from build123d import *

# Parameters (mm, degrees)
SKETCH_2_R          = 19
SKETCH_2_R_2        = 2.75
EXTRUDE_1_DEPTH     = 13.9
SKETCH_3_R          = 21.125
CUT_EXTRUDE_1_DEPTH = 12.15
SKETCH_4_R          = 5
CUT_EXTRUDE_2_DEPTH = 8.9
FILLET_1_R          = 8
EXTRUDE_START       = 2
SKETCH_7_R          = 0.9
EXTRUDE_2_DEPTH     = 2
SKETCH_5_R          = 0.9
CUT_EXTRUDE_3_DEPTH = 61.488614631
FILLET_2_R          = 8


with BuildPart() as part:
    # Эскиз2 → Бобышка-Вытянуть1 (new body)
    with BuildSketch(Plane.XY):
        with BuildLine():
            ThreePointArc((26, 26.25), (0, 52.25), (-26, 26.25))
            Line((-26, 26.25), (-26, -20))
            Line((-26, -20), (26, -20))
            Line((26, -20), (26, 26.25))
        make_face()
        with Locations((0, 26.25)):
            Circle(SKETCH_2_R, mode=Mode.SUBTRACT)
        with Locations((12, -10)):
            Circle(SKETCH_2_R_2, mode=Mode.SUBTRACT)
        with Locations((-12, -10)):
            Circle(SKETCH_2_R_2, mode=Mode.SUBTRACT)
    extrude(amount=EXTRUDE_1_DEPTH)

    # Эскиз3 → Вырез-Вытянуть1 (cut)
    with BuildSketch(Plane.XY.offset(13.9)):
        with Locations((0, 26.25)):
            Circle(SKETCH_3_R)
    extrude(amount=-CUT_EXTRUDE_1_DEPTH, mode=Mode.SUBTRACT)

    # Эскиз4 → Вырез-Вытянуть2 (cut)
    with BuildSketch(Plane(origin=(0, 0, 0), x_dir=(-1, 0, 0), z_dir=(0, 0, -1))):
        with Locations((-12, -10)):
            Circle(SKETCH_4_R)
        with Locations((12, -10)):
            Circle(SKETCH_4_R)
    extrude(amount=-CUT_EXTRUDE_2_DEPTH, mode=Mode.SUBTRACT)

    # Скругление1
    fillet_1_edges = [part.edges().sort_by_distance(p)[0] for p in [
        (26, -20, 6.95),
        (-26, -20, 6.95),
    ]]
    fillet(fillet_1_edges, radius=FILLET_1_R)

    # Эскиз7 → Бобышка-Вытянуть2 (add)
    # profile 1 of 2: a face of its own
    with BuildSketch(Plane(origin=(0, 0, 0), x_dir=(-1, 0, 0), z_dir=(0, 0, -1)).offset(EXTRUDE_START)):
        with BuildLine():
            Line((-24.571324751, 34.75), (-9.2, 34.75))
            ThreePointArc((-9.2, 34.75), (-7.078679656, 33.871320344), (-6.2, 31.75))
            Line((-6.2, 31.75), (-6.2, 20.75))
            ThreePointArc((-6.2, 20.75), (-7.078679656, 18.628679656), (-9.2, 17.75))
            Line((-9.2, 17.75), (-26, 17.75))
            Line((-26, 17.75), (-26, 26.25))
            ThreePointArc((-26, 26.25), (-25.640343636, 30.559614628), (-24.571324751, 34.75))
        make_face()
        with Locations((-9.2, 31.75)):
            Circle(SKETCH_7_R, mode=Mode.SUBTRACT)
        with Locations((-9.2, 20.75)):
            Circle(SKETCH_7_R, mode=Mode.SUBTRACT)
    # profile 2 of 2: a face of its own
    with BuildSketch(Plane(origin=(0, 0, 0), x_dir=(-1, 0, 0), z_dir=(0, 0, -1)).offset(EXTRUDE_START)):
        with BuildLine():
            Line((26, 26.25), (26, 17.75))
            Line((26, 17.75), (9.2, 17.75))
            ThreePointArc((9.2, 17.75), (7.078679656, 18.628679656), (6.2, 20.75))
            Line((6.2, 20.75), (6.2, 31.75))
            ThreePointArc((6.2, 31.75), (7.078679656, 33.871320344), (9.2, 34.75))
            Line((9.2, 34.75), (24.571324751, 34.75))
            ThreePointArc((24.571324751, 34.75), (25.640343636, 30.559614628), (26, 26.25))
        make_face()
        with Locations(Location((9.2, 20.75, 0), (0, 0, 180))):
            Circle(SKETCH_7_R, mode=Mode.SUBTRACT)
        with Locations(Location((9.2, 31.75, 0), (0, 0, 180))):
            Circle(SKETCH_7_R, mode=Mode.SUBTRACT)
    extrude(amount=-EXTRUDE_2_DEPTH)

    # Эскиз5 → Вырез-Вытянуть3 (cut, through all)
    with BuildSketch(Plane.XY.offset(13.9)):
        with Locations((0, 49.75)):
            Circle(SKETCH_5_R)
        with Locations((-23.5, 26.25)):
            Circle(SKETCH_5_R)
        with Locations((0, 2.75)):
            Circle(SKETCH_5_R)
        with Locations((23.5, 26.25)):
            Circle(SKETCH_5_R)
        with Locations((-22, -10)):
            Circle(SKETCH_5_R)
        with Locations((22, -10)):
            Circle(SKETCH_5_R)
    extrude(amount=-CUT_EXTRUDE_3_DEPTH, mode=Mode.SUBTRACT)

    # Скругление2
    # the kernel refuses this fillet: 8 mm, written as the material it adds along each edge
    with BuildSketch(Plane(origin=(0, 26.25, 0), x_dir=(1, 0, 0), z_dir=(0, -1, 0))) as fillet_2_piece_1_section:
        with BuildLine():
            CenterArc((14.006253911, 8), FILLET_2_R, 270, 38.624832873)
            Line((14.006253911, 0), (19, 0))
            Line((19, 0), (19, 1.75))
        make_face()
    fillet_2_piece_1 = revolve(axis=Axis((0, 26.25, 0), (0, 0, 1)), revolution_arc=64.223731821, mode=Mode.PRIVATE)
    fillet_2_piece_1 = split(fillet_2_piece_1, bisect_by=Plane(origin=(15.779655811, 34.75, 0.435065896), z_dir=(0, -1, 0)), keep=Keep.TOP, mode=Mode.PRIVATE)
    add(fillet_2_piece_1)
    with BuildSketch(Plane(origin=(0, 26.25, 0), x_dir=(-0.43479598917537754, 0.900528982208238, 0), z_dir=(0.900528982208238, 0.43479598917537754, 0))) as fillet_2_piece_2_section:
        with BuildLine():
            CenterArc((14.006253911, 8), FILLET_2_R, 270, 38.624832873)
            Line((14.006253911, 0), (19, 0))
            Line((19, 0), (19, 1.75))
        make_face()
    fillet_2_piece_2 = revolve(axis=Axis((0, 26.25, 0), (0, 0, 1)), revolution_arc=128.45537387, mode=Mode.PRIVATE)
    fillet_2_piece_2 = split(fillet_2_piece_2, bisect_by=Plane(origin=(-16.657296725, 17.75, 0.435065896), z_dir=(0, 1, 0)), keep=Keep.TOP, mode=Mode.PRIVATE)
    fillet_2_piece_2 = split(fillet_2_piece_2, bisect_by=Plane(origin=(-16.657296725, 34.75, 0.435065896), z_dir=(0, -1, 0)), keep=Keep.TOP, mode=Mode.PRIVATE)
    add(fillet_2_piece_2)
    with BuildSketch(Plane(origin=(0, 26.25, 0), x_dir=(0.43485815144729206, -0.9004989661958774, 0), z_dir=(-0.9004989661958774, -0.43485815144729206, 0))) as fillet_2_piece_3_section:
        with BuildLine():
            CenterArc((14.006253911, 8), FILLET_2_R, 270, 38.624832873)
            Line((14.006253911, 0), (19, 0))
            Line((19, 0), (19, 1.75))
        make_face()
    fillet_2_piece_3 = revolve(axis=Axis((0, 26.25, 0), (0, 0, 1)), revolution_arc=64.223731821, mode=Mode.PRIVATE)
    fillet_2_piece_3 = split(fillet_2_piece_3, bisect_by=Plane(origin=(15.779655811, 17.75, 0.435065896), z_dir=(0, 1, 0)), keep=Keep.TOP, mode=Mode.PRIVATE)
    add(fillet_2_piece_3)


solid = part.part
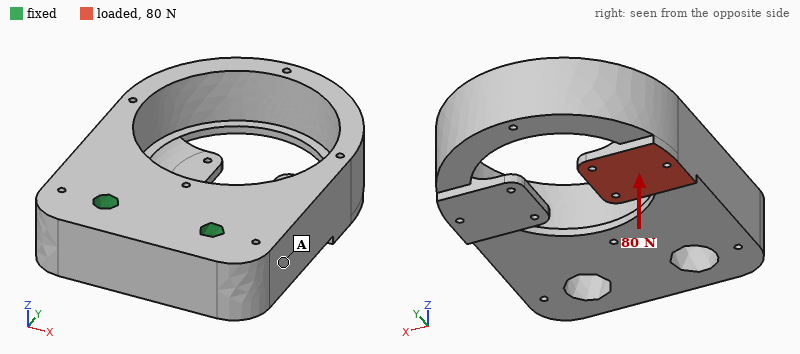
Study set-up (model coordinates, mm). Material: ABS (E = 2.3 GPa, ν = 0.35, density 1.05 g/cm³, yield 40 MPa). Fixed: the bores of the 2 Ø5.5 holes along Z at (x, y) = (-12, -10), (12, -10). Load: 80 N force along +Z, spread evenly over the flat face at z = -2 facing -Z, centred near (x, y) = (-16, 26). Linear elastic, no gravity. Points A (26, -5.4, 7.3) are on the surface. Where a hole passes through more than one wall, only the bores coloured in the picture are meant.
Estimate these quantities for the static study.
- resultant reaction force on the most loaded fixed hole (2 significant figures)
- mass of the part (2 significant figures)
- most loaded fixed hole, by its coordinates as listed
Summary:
88 N
30 g
(-12, -10)
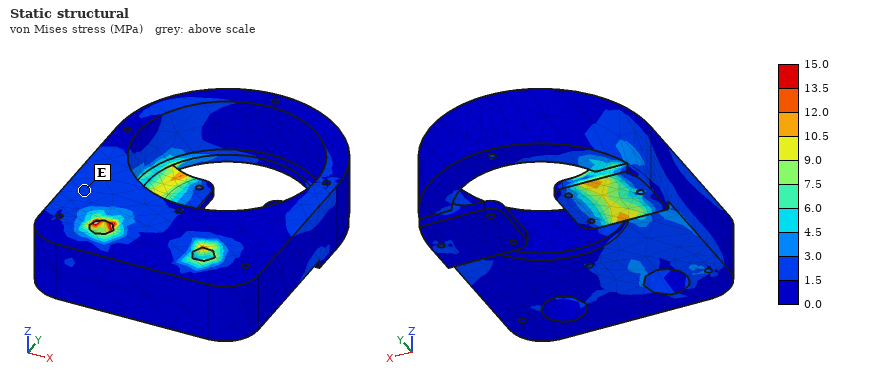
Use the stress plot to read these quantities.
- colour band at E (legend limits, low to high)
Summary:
1.5 to 3.0 MPa
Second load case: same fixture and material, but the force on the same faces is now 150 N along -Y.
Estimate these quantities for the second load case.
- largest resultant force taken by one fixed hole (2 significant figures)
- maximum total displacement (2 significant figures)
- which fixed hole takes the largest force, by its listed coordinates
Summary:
160 N
0.42 mm
(-12, -10)
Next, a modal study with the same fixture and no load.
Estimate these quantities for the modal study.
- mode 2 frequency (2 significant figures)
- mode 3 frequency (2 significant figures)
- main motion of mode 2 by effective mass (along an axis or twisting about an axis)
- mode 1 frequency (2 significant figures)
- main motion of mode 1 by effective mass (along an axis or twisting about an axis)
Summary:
1100 Hz
1600 Hz
along X
660 Hz
along Z
